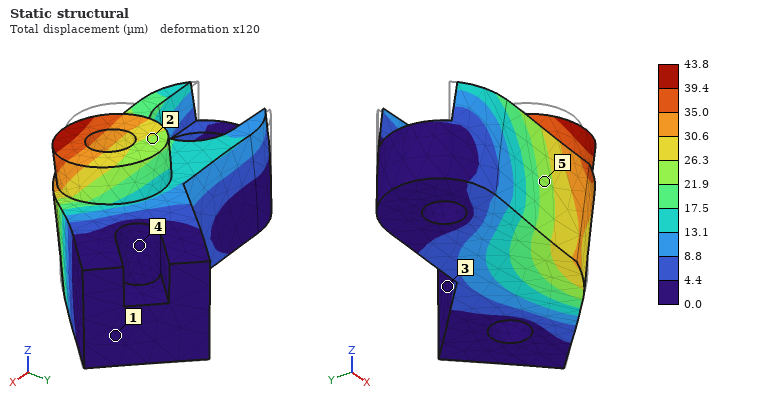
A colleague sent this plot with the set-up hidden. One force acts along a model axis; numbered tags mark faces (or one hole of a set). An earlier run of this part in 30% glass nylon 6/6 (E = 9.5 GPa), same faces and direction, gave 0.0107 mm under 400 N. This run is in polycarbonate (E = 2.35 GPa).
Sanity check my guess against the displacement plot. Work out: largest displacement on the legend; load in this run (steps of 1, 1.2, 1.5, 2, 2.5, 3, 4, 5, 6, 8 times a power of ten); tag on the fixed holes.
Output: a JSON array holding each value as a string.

["43.8 µm", "400 N", "4"]
